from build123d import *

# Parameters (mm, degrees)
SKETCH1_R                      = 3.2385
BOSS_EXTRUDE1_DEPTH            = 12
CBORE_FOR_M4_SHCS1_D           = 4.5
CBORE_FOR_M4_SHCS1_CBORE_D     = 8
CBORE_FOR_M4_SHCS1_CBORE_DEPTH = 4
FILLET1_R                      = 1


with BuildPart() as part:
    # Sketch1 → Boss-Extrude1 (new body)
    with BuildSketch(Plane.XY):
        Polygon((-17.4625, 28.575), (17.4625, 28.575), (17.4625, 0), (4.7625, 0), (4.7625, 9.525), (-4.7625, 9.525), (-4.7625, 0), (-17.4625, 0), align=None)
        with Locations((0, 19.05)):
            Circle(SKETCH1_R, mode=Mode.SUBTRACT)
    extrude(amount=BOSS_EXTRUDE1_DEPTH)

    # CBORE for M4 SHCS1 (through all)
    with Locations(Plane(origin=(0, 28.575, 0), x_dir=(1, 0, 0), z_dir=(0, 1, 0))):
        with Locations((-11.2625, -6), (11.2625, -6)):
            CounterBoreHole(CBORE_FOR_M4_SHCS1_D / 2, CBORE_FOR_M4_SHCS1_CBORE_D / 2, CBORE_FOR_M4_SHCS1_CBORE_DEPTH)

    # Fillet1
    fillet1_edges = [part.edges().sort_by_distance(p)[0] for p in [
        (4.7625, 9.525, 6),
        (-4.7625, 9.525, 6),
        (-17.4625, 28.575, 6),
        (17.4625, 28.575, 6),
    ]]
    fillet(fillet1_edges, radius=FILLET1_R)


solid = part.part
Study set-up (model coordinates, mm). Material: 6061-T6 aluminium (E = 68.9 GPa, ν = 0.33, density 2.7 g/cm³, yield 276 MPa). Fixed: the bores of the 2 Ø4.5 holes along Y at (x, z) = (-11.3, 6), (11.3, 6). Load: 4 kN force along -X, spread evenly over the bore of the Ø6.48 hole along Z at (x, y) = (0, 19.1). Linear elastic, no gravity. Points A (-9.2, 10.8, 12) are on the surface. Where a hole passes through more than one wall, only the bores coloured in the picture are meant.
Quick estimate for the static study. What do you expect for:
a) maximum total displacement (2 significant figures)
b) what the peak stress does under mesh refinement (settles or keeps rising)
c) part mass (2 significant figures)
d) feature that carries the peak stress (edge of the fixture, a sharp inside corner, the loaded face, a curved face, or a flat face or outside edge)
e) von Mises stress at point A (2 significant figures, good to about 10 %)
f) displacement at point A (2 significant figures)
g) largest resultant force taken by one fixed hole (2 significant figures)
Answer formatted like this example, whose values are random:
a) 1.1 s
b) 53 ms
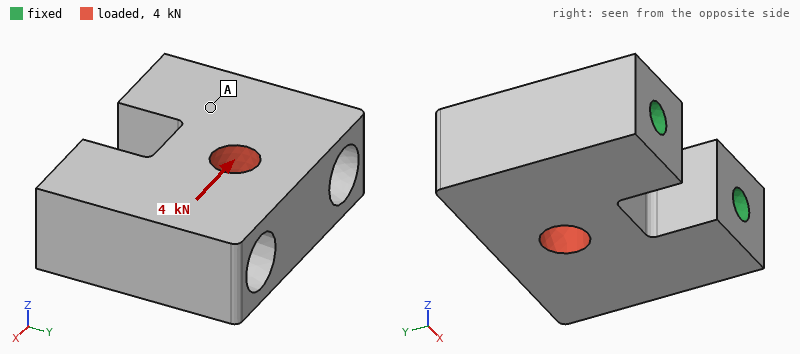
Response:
a) 2.3 µm
b) keeps rising
c) 25 g
d) edge of the fixture
e) 3.9 MPa
f) 0.36 µm
g) 2.0 kN
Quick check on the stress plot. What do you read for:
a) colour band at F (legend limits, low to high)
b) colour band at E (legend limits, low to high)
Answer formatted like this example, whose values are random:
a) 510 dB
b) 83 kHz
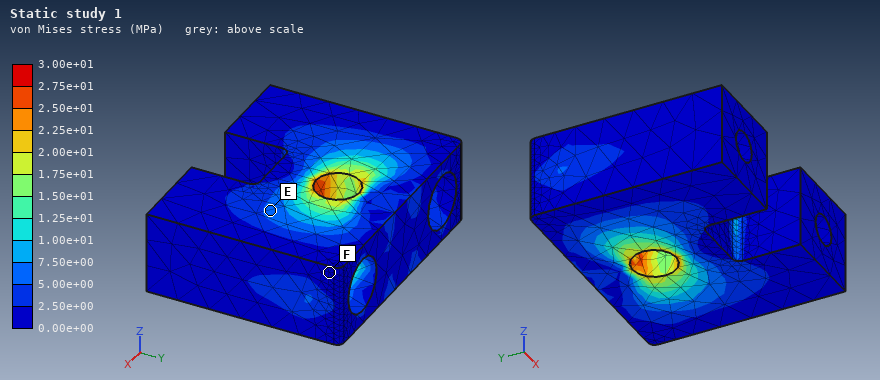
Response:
a) 0.00e+00 to 2.50e+00 MPa
b) 5.00e+00 to 7.50e+00 MPa
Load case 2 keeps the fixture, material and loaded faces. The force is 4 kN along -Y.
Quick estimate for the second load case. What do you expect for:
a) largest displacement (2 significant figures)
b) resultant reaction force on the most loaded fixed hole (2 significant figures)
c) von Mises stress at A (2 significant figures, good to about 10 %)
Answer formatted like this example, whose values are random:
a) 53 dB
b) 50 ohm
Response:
a) 4.4 µm
b) 2.1 kN
c) 6.3 MPa
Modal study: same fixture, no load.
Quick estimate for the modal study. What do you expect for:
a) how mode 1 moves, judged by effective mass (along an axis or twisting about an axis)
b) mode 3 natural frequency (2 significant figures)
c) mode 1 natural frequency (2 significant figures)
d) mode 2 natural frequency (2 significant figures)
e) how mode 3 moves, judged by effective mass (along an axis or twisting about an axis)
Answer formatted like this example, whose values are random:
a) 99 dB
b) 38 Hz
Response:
a) along Z
b) 71 kHz
c) 46 kHz
d) 65 kHz
e) along Y
